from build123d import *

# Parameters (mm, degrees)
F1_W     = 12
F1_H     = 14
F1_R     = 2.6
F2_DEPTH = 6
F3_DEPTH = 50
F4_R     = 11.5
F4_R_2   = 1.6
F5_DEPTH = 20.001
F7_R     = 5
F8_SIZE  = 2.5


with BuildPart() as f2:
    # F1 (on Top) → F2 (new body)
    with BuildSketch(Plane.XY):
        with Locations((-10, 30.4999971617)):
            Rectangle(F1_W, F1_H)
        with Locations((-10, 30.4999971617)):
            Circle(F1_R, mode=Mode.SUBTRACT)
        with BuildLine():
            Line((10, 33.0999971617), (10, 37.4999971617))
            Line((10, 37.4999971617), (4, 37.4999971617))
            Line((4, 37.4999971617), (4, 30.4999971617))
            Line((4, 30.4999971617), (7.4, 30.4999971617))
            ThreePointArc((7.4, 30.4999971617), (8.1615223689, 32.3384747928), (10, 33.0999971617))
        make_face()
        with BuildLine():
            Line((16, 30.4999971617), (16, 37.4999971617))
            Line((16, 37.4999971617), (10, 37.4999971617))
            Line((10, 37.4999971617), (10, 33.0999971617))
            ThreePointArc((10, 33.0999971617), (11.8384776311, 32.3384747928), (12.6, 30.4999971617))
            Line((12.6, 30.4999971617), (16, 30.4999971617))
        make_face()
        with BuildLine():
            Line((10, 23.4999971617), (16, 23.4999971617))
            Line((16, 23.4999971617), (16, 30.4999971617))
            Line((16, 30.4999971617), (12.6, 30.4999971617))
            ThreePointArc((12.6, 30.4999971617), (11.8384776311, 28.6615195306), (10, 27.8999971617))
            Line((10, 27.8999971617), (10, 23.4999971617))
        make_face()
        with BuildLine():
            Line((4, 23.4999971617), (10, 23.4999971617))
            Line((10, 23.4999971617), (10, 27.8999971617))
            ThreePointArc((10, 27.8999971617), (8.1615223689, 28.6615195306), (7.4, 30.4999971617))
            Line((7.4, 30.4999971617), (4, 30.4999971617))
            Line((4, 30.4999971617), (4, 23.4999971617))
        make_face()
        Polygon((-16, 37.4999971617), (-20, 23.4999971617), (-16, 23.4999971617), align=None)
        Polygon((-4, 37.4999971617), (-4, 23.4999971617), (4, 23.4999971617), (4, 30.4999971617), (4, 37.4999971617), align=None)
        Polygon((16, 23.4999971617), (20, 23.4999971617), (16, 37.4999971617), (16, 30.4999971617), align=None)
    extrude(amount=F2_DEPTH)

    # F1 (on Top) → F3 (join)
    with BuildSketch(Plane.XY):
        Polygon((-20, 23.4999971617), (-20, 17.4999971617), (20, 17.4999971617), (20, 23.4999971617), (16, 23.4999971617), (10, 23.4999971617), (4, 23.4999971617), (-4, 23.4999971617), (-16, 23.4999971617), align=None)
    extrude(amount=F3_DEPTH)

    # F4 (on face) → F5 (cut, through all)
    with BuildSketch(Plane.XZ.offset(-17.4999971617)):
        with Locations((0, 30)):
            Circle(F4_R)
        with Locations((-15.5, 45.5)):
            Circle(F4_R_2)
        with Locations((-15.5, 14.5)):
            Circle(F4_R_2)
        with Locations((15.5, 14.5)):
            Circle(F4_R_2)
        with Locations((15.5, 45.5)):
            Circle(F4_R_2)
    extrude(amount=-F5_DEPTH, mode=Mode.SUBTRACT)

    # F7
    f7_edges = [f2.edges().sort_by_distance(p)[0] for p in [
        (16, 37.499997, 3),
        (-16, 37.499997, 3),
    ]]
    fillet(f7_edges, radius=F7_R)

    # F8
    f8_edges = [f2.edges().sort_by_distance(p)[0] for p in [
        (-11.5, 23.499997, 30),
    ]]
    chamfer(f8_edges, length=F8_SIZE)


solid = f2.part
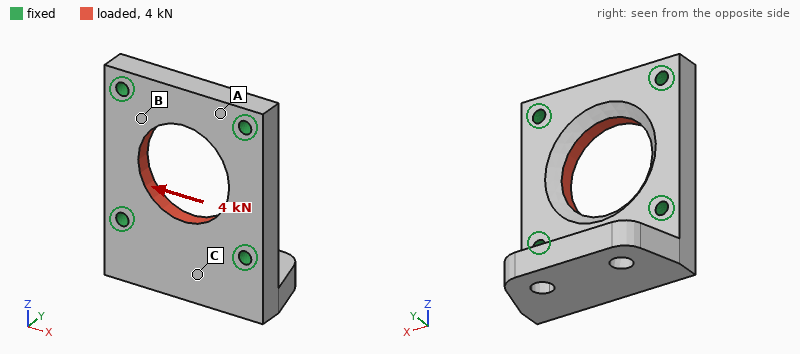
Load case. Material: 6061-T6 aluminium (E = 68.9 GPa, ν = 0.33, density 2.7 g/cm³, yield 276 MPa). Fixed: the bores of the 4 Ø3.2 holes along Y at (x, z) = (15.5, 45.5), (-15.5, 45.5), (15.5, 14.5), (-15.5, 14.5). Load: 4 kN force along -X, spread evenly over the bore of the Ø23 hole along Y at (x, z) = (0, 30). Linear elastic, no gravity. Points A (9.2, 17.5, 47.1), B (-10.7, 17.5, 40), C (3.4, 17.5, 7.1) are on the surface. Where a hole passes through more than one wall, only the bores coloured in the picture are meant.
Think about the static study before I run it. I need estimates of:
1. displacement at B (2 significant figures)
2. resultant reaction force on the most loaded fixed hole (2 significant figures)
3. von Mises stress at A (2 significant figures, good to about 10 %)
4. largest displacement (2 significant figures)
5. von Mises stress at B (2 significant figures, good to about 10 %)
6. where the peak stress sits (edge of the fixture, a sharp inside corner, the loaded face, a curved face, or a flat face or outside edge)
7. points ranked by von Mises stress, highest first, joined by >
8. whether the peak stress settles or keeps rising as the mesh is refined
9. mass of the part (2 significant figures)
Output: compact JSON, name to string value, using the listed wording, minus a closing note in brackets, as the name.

{"displacement at B": "3.5 µm", "resultant reaction force on the most loaded fixed hole": "1.1 kN", "von Mises stress at A": "12 MPa", "largest displacement": "9.3 µm", "von Mises stress at B": "21 MPa", "where the peak stress sits": "edge of the fixture", "points ranked by von Mises stress, highest first, joined by >": "B > A > C", "whether the peak stress settles or keeps rising as the mesh is refined": "keeps rising", "mass of the part": "32 g"}
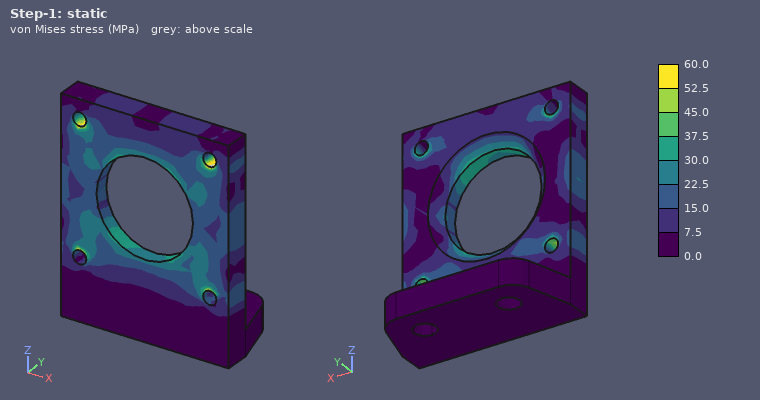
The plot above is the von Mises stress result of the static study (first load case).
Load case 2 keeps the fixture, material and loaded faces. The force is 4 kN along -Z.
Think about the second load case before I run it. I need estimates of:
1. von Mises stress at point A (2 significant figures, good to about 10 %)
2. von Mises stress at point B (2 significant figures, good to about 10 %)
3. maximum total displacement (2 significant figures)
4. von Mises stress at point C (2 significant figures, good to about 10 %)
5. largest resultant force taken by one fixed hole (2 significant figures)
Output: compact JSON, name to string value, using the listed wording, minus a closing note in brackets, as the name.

{"von Mises stress at point A": "20 MPa", "von Mises stress at point B": "19 MPa", "maximum total displacement": "10 µm", "von Mises stress at point C": "6.0 MPa", "largest resultant force taken by one fixed hole": "1.0 kN"}
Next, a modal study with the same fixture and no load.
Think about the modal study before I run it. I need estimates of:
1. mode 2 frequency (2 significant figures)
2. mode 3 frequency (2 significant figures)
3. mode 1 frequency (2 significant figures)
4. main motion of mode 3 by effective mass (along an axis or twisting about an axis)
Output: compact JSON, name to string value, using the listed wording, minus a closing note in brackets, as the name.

{"mode 2 frequency": "14 kHz", "mode 3 frequency": "18 kHz", "mode 1 frequency": "7500 Hz", "main motion of mode 3 by effective mass": "along Y"}
